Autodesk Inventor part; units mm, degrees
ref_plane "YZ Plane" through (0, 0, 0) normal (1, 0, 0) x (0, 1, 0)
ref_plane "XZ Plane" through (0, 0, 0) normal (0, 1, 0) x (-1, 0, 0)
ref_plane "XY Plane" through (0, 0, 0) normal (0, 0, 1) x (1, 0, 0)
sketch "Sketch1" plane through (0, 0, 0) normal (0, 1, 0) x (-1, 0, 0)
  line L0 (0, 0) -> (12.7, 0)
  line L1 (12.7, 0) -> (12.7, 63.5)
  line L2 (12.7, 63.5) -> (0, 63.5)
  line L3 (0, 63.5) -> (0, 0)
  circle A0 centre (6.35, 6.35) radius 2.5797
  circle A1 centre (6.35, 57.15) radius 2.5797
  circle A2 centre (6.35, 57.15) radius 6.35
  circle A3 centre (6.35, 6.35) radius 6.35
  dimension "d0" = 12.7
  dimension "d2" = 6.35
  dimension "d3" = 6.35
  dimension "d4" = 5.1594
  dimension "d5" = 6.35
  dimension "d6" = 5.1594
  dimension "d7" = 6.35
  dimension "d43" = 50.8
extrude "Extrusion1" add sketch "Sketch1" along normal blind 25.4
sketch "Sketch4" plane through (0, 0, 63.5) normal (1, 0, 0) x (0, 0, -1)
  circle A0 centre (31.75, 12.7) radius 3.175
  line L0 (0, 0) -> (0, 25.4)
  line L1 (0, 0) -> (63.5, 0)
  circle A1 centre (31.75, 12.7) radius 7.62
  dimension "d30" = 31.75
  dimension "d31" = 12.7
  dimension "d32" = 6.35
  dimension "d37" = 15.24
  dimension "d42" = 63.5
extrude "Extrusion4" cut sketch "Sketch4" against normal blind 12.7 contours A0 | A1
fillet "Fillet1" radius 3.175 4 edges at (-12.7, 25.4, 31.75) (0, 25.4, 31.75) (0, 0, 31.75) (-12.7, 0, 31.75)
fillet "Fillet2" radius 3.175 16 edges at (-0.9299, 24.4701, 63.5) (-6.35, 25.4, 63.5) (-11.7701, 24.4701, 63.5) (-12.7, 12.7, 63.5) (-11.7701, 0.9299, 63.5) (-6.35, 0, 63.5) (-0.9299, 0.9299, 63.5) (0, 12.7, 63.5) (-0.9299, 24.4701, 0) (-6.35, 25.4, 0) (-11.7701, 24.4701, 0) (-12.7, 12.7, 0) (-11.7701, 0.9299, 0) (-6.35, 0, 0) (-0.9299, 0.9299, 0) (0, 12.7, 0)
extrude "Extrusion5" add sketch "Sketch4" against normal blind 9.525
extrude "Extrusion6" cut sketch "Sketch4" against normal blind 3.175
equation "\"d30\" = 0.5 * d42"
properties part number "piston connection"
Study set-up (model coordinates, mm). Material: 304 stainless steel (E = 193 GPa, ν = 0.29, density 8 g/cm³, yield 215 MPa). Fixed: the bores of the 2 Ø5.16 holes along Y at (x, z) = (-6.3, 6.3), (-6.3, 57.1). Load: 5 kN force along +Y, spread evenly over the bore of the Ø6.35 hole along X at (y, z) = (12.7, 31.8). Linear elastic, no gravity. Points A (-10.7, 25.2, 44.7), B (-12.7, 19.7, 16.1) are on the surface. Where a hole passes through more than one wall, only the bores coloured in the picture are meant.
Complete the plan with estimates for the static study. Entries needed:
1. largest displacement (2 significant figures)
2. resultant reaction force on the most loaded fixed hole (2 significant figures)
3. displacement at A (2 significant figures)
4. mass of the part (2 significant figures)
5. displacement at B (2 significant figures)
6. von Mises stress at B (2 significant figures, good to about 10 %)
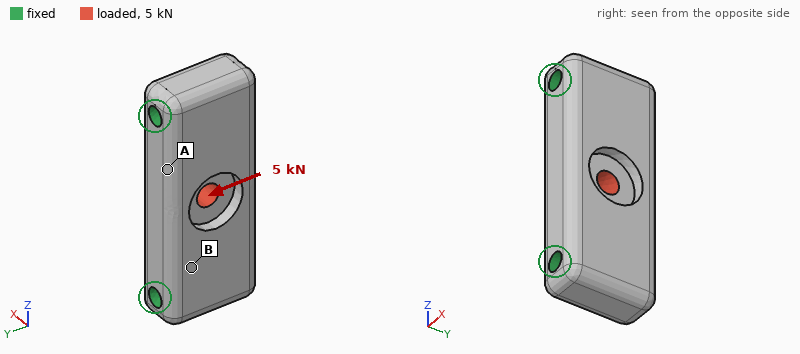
4.7 µm
2.5 kN
2.0 µm
140 g
1.3 µm
15 MPa
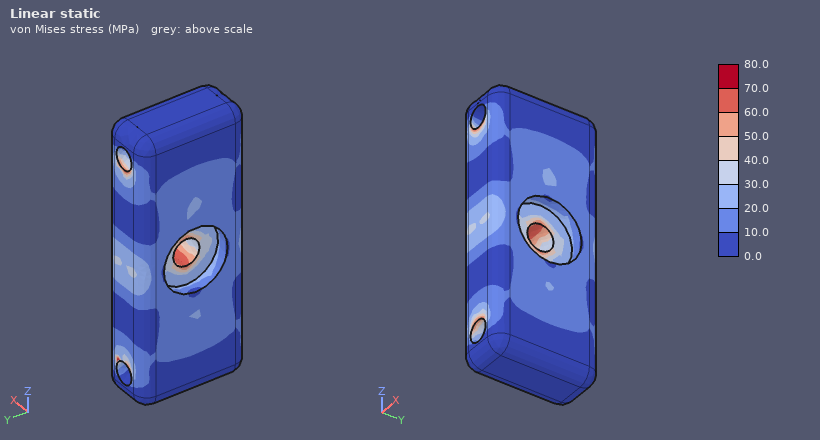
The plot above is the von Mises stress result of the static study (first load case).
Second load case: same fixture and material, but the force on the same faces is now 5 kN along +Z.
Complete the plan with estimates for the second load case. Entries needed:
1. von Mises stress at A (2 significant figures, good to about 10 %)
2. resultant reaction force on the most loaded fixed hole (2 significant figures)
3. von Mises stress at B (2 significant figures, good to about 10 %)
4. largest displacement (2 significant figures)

5.4 MPa
2.5 kN
7.4 MPa
2.0 µm
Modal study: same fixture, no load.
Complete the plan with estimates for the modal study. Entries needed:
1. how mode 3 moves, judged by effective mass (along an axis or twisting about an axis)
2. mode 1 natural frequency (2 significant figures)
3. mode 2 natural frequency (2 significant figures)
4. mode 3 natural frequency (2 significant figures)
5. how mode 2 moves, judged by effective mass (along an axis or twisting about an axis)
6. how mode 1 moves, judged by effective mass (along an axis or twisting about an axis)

along Y
17 kHz
26 kHz
28 kHz
twisting about Z
along X
